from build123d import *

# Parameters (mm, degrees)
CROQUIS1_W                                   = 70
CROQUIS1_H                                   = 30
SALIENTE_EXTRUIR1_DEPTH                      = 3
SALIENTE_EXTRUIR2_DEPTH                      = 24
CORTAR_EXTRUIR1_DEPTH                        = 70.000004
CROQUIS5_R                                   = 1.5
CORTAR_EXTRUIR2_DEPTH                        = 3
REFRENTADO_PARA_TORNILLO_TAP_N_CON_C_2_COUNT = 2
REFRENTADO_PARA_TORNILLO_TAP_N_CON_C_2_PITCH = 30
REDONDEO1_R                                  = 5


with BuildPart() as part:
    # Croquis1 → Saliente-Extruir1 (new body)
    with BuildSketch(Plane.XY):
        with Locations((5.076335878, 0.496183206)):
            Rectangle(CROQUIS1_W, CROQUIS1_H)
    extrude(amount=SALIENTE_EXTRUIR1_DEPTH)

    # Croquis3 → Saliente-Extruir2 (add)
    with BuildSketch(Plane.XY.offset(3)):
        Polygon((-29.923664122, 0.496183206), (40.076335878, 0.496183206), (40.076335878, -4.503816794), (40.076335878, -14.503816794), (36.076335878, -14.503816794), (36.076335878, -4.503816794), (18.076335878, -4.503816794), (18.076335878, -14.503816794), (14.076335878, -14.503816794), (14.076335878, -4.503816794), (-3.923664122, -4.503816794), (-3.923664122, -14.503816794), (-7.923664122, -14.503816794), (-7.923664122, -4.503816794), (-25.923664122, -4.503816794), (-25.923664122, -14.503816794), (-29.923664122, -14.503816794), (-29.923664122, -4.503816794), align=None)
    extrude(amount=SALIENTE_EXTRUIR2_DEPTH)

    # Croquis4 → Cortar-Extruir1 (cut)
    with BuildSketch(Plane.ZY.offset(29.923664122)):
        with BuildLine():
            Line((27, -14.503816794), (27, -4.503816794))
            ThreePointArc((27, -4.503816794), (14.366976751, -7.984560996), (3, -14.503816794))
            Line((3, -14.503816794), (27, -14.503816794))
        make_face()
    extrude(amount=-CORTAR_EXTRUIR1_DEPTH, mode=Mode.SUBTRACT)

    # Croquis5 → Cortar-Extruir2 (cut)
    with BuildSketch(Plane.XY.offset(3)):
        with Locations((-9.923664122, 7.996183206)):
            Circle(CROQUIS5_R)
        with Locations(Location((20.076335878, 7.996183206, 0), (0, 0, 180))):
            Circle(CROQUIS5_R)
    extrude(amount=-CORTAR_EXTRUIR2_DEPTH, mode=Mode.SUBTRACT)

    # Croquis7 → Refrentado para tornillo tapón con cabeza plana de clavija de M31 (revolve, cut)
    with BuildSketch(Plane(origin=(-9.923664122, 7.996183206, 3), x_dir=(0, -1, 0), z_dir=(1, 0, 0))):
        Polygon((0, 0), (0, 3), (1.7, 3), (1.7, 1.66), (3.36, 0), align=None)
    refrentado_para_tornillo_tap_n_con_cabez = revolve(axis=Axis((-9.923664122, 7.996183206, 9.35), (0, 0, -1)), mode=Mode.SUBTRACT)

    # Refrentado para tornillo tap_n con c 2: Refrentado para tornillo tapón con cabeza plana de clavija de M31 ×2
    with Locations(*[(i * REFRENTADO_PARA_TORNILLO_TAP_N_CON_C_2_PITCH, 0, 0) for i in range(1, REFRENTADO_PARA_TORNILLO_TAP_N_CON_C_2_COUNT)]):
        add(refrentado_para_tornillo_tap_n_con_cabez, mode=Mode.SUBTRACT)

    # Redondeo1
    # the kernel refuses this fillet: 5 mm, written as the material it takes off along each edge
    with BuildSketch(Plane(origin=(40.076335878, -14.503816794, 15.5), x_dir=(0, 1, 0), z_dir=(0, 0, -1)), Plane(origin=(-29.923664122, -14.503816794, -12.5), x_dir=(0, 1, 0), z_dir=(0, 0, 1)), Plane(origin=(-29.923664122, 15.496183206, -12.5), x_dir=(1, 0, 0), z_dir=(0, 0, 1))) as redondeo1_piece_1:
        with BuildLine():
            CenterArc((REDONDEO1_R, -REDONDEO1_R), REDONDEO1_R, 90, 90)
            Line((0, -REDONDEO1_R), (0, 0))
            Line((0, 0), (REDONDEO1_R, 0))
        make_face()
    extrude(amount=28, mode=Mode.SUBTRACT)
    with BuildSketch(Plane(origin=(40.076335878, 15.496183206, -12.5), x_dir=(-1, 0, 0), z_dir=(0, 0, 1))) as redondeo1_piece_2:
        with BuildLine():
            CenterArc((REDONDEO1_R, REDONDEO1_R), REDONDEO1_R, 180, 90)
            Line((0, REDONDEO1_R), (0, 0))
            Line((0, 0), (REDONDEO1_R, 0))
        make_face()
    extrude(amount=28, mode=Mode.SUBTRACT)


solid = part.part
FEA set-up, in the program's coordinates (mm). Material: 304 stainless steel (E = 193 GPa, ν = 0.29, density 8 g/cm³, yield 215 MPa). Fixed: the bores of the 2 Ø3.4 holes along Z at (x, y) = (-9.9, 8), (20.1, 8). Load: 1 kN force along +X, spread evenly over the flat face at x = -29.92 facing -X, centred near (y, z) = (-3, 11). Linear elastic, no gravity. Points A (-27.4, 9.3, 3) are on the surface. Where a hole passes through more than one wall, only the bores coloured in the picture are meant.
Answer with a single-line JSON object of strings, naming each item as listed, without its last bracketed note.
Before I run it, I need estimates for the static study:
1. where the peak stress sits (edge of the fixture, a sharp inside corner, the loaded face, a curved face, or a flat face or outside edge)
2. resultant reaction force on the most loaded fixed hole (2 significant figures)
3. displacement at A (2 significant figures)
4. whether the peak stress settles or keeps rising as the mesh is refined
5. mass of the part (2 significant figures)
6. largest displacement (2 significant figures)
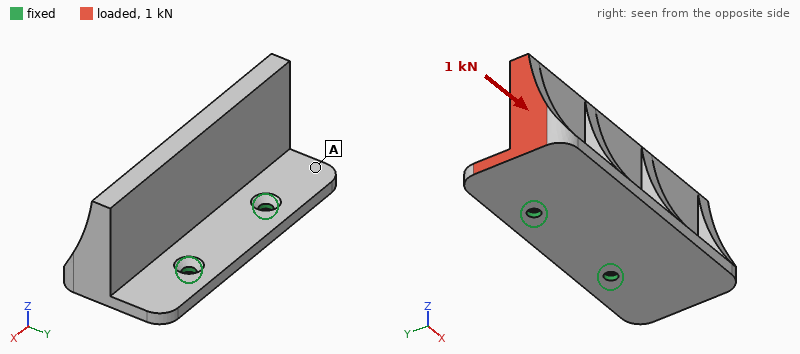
{"where the peak stress sits": "edge of the fixture", "resultant reaction force on the most loaded fixed hole": "710 N", "displacement at A": "8.6 µm", "whether the peak stress settles or keeps rising as the mesh is refined": "keeps rising", "mass of the part": "130 g", "largest displacement": "18 µm"}
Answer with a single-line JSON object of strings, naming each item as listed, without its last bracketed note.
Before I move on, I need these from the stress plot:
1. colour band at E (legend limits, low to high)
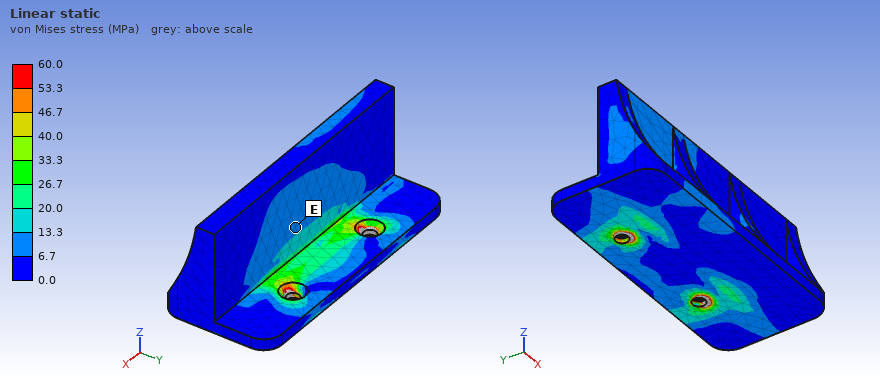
{"colour band at E": "6.7 to 13.3 MPa"}
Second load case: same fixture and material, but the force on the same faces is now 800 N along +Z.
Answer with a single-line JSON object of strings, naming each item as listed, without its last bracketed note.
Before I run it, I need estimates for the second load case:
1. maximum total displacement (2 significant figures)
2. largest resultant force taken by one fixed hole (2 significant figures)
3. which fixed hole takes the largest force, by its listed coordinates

{"maximum total displacement": "0.17 mm", "largest resultant force taken by one fixed hole": "1.3 kN", "which fixed hole takes the largest force, by its listed coordinates": "(-9.9, 8)"}
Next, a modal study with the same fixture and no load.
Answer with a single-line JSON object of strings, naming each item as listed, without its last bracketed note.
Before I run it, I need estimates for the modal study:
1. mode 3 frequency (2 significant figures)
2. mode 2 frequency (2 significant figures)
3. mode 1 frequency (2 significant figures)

{"mode 3 frequency": "5400 Hz", "mode 2 frequency": "2800 Hz", "mode 1 frequency": "1200 Hz"}
